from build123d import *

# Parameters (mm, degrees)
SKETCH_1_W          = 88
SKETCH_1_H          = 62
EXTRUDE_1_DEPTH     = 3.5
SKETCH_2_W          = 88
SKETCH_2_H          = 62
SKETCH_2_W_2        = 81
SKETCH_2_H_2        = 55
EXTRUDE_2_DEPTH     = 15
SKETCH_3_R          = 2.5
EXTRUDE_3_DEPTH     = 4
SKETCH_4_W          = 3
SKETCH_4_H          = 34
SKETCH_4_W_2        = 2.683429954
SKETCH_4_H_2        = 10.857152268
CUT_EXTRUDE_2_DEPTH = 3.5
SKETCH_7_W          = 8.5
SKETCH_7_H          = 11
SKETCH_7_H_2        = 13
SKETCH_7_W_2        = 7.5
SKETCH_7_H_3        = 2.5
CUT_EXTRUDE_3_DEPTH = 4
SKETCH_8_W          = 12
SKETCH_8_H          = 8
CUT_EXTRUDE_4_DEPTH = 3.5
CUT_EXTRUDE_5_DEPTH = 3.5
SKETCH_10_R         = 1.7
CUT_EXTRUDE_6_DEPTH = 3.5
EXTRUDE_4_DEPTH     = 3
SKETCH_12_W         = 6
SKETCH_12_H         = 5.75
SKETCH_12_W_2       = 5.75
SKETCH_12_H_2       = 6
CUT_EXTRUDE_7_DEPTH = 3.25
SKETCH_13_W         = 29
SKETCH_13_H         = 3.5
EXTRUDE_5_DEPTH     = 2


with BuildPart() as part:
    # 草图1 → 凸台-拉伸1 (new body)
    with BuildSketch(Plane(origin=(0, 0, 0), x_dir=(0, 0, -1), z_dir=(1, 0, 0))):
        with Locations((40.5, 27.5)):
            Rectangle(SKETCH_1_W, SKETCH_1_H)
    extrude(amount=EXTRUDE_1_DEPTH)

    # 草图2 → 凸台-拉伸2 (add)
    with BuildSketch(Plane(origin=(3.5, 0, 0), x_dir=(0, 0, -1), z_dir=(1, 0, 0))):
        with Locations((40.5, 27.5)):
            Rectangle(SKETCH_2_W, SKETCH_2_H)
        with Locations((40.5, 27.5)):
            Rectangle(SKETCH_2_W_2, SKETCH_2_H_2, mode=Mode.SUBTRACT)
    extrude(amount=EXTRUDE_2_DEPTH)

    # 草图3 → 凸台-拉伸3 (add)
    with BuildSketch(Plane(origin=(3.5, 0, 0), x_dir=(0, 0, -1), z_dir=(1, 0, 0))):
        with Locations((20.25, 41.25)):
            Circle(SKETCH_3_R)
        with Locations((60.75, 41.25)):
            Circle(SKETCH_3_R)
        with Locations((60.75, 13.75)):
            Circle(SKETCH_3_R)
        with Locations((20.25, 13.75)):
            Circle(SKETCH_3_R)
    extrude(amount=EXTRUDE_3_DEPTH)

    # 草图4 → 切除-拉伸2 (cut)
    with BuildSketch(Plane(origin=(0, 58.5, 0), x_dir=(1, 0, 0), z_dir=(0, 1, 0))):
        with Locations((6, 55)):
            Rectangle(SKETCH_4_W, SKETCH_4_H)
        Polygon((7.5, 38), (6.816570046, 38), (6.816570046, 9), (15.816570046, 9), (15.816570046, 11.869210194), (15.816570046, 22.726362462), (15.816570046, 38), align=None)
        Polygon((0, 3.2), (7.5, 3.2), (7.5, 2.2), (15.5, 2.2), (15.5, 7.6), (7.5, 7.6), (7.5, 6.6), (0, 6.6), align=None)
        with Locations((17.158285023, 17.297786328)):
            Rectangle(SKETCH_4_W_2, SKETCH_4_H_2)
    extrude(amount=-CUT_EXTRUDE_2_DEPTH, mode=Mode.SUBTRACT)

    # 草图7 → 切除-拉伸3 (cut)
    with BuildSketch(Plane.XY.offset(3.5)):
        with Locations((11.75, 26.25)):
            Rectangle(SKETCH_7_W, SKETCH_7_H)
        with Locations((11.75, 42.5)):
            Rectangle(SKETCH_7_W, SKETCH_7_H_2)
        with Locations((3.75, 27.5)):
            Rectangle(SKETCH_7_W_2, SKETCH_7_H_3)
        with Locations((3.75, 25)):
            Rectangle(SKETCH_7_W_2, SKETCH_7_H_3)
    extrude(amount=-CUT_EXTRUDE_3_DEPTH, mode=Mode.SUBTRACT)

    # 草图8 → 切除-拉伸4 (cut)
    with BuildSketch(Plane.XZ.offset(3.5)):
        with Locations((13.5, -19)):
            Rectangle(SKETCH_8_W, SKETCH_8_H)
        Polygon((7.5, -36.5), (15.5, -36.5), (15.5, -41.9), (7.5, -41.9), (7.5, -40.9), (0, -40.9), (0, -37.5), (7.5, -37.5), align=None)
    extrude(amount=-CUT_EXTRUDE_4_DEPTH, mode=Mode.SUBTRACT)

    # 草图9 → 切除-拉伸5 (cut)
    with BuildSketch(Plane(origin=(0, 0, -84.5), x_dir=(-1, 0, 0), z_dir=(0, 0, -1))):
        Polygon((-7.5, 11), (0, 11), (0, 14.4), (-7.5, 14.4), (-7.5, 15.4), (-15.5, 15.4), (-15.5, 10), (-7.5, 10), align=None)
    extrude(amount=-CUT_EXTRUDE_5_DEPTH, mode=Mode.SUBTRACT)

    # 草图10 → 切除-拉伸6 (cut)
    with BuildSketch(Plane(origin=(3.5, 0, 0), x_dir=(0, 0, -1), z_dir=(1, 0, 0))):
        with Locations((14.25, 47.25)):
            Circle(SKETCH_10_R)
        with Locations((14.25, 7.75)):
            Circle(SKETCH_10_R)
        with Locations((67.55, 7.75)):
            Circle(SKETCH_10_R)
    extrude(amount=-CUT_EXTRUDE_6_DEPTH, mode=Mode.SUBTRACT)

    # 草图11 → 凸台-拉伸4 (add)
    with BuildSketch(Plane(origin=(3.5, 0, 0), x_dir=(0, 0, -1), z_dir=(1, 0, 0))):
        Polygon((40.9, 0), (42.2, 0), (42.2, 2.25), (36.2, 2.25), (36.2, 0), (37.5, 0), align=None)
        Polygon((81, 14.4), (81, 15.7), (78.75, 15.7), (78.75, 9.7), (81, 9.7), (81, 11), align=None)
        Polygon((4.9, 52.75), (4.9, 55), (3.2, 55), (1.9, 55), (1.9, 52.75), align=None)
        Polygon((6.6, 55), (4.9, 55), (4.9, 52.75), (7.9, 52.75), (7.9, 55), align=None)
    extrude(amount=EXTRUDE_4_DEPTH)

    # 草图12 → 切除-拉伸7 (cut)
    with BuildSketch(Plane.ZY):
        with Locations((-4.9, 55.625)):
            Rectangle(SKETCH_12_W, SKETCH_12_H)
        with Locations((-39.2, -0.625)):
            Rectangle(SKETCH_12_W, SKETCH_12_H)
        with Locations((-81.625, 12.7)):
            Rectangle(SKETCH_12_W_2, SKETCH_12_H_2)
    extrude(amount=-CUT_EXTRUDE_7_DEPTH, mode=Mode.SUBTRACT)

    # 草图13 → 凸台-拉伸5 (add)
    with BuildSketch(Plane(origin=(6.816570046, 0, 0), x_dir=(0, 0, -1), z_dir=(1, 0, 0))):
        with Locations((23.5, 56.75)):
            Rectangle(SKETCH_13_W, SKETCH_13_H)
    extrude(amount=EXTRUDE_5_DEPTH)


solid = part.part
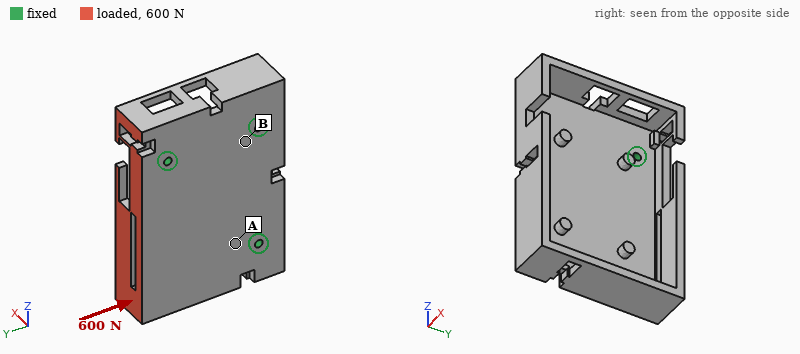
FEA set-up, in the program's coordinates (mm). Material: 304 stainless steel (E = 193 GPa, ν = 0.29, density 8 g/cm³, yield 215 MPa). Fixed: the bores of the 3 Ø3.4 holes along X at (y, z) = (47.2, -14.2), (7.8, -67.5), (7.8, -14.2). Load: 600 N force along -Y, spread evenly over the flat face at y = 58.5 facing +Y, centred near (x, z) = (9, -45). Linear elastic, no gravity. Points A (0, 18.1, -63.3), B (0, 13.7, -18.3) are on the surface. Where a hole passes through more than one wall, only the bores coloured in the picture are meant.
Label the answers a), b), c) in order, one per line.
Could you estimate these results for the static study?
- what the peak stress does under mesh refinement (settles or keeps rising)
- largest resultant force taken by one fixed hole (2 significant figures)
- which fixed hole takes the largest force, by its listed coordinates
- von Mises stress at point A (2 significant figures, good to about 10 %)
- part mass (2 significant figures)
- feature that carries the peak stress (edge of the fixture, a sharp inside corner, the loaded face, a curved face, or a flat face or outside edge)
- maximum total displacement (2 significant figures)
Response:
a) keeps rising
b) 330 N
c) (7.8, -67.5)
d) 9.5 MPa
e) 250 g
f) a sharp inside corner
g) 43 µm
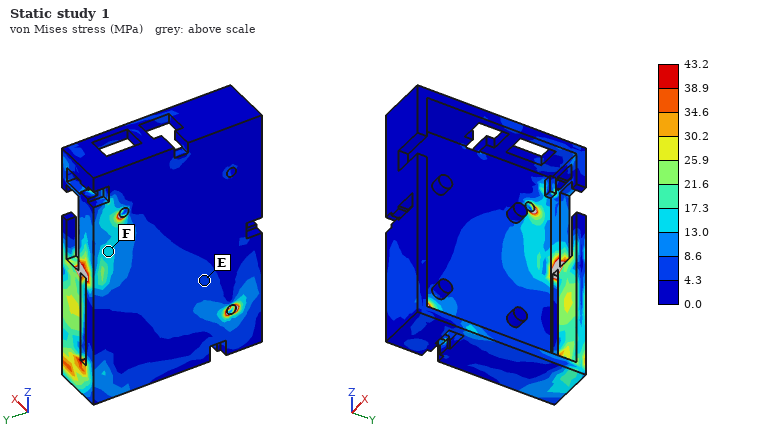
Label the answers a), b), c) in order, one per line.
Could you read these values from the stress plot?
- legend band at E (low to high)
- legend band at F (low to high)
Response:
a) 4.3 to 8.6 MPa
b) 13.0 to 17.3 MPa
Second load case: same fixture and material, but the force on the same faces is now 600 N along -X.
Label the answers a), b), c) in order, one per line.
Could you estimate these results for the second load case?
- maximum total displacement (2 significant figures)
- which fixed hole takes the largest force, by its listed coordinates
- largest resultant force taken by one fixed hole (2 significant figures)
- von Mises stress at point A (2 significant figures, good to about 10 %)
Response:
a) 0.17 mm
b) (47.2, -14.2)
c) 530 N
d) 50 MPa
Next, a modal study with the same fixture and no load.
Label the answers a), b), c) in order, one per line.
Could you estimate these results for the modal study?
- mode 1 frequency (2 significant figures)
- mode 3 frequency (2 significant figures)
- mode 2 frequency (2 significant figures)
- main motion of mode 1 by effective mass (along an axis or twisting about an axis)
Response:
a) 1200 Hz
b) 4400 Hz
c) 3900 Hz
d) along X
